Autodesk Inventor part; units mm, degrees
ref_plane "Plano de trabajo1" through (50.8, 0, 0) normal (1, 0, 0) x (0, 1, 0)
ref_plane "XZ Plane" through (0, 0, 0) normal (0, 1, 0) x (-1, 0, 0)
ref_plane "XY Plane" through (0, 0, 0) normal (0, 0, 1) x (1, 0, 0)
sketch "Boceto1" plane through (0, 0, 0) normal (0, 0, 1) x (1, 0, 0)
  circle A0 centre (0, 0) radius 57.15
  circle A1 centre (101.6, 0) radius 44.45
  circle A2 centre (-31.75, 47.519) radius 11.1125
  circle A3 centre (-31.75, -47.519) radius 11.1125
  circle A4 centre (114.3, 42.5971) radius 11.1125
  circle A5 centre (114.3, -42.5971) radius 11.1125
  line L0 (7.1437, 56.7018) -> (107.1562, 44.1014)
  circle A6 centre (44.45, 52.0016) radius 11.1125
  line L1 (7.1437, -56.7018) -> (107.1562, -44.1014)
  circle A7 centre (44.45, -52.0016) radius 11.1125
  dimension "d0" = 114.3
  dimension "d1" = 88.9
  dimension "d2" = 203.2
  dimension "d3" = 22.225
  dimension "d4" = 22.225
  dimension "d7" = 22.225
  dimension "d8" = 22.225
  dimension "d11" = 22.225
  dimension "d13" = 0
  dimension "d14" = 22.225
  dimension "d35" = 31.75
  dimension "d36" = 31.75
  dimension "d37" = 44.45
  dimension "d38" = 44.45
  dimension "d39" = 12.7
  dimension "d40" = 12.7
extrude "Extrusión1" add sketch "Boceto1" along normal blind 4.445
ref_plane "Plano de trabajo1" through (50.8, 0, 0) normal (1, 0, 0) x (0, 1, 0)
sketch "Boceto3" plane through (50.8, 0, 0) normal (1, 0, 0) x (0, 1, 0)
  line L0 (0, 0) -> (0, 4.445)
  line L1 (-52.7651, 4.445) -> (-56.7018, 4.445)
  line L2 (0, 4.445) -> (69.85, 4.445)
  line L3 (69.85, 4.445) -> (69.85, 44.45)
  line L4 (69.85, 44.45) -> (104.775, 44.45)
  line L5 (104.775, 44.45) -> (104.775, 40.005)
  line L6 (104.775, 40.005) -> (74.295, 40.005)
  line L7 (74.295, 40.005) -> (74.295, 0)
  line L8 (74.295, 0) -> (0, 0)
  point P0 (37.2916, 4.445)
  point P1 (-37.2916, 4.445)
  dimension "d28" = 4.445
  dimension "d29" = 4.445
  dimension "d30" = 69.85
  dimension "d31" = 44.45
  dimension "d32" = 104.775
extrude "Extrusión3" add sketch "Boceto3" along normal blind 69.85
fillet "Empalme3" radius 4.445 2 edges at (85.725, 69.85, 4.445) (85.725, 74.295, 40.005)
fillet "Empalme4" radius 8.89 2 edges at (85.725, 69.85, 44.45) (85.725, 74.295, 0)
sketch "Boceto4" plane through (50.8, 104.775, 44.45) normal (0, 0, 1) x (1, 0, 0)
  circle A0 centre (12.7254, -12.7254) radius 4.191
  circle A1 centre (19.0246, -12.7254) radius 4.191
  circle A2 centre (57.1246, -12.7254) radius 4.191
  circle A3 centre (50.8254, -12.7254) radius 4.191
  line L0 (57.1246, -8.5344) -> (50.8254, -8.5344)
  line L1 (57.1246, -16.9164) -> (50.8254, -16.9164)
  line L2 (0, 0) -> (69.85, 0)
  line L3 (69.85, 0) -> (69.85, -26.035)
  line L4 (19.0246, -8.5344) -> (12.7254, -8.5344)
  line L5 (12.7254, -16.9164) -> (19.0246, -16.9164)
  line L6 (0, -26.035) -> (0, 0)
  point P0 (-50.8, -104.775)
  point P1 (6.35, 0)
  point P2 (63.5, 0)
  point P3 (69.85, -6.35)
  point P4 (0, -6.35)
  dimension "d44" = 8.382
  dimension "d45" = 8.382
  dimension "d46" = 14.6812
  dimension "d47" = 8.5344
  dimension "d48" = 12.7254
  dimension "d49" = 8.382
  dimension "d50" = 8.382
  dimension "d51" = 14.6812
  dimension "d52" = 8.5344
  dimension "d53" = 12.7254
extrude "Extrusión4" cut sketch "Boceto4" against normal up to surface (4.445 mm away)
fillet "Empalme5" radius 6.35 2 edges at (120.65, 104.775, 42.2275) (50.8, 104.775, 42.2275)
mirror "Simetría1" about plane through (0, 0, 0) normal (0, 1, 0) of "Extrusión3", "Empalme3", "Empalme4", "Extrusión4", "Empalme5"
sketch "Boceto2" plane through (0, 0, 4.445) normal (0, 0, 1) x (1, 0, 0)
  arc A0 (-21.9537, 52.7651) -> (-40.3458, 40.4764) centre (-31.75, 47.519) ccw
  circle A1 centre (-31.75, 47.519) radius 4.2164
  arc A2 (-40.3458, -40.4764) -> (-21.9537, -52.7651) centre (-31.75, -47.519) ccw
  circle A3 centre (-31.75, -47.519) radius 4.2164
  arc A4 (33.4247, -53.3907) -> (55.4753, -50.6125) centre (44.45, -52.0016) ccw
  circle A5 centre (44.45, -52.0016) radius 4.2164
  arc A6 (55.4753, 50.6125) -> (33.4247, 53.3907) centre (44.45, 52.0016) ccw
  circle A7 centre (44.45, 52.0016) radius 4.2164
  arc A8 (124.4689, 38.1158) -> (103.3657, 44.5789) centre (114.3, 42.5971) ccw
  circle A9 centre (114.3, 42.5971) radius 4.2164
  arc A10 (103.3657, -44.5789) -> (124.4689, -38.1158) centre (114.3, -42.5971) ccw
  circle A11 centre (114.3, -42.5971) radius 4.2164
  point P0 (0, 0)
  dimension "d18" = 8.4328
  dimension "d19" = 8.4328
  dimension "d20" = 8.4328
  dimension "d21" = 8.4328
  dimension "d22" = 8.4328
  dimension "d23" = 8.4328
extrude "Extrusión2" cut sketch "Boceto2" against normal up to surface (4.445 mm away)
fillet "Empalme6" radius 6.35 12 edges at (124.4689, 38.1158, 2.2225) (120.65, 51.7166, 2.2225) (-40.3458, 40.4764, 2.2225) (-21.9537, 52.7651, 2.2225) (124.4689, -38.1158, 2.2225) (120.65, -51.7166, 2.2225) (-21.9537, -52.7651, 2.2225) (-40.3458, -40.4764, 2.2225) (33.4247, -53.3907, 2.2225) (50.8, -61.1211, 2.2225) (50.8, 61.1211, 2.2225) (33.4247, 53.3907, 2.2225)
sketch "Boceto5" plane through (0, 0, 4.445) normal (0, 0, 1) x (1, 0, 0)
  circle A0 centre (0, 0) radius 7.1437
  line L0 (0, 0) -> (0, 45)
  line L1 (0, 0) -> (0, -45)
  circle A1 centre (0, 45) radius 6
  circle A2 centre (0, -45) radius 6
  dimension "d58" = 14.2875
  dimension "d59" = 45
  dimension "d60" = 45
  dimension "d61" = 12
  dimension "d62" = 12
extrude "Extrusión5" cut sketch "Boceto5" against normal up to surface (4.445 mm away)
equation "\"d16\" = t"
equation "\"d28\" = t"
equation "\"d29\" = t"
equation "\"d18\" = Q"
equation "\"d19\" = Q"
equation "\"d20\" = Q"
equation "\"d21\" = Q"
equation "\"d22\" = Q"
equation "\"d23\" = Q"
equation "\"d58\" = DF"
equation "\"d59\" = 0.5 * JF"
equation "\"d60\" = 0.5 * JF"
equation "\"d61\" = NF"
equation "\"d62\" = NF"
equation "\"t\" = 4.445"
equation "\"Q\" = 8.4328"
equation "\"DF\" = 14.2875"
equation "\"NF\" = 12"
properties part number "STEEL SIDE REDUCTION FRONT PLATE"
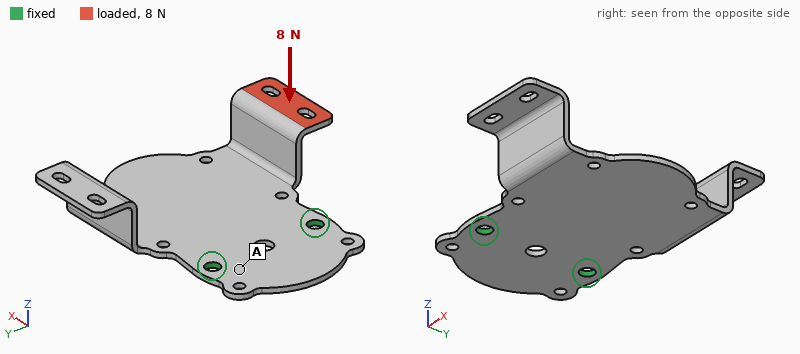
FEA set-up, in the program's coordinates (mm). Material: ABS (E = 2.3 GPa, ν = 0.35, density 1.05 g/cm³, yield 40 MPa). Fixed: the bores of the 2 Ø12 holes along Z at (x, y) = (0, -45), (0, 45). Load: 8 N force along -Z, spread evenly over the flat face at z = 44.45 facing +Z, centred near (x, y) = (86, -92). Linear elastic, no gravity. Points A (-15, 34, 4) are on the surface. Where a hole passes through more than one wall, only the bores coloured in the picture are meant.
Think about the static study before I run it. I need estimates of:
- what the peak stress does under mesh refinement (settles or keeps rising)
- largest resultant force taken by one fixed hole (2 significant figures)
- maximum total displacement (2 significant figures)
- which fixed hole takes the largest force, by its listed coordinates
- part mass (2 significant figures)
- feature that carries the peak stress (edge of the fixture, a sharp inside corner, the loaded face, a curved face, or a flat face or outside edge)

keeps rising
12 N
3.4 mm
(0, -45)
150 g
edge of the fixture
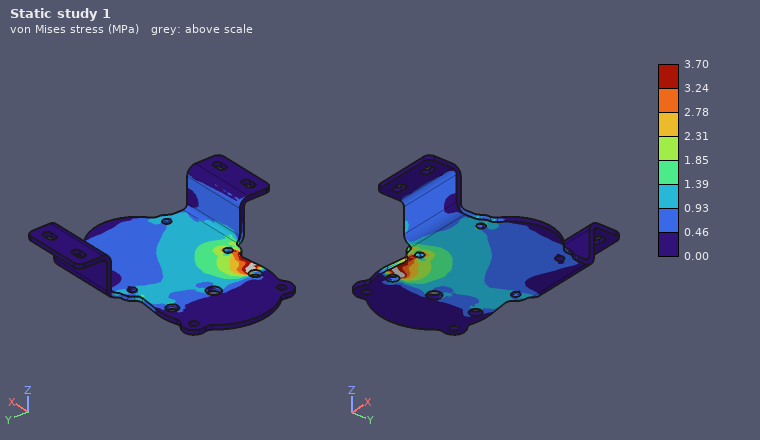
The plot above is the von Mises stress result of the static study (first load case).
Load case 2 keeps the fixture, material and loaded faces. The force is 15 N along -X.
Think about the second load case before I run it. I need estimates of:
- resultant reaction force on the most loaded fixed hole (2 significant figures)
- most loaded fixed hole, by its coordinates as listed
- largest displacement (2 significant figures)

23 N
(0, -45)
3.2 mm
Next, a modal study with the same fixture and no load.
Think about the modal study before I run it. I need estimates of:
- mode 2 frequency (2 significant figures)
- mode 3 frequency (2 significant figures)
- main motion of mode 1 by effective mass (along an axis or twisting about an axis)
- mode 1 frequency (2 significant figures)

65 Hz
120 Hz
along Z
41 Hz
